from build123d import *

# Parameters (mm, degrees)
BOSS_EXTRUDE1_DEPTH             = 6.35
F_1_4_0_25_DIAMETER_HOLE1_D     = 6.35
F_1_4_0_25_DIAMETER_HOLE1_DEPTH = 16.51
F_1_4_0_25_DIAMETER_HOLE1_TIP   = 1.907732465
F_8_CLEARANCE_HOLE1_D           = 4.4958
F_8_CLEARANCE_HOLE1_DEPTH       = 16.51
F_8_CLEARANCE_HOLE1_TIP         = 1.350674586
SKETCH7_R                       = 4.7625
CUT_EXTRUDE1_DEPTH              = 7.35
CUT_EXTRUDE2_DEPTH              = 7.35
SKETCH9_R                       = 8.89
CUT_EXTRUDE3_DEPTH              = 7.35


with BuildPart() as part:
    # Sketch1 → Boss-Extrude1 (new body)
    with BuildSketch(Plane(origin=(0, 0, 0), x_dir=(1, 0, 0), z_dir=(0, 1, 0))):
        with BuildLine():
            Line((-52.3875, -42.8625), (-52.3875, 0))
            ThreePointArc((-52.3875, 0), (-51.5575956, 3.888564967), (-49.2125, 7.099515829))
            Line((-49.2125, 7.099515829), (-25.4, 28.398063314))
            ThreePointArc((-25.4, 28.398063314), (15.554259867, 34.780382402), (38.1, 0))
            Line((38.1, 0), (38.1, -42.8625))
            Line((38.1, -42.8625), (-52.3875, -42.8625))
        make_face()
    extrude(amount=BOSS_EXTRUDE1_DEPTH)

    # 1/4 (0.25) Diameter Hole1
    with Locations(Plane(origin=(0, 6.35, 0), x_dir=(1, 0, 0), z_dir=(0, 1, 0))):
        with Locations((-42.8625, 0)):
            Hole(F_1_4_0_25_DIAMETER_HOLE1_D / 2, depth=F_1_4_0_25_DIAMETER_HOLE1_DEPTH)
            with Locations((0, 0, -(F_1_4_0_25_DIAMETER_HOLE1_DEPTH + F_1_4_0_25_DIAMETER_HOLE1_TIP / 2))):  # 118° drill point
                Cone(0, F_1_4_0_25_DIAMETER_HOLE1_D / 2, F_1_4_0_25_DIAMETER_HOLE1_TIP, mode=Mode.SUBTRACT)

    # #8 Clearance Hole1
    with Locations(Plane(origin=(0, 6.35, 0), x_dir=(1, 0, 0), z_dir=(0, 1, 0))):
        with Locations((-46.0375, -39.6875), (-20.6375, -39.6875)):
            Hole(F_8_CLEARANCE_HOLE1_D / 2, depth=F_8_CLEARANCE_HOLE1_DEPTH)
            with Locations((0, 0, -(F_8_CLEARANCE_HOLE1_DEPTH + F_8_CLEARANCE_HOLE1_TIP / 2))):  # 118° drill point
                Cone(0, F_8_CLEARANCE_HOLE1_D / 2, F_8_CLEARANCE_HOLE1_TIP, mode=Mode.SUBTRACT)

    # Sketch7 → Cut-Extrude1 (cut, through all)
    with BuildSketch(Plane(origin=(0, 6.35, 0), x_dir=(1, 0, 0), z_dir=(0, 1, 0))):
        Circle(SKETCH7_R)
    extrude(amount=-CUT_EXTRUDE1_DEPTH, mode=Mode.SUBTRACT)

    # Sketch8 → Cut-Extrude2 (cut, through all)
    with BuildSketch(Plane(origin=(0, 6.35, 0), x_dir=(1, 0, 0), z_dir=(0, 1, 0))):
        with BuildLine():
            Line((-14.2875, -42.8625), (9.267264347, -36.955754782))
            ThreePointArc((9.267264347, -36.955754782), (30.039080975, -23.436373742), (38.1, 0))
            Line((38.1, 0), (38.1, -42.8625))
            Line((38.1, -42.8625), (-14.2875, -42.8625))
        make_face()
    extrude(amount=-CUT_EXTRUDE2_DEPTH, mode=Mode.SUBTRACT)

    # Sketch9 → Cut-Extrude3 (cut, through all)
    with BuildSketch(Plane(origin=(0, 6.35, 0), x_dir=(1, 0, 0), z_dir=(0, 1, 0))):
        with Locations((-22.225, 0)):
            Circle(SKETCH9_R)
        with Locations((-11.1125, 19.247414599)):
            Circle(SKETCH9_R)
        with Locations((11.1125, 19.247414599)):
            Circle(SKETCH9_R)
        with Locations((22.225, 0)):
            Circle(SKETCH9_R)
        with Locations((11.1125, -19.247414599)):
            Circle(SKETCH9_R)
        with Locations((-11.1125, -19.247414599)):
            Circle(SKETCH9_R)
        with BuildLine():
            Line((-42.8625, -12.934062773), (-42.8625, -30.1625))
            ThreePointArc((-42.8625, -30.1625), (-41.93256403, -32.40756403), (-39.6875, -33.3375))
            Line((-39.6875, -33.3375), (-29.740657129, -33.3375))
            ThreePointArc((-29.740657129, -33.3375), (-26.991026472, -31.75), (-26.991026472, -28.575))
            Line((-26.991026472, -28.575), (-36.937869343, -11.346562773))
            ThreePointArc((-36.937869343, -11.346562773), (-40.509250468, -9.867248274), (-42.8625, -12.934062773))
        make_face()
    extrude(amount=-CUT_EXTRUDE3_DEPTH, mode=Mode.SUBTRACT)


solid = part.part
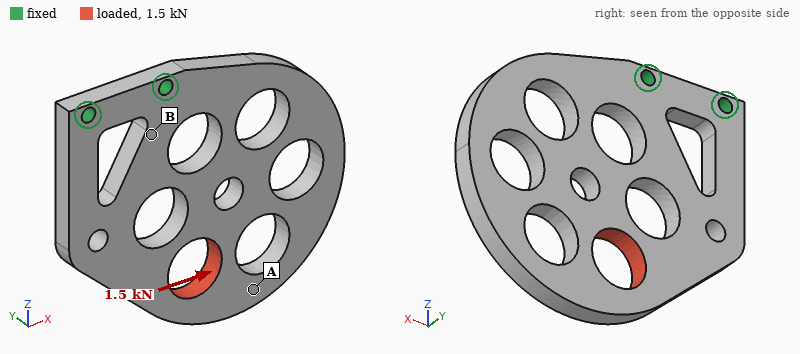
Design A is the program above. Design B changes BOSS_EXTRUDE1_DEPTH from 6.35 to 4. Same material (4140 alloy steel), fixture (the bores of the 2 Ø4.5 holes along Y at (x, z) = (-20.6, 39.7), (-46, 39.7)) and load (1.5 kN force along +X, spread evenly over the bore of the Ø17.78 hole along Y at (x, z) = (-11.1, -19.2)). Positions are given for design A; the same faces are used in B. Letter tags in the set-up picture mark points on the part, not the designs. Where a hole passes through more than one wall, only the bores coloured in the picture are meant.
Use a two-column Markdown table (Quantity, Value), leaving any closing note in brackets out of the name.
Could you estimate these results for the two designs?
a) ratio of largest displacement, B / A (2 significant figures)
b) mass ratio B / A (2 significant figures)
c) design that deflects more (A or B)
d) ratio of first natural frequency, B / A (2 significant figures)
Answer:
| Quantity | Value |
|---|---|
| ratio of largest displacement, B / A | 1.6 |
| mass ratio B / A | 0.63 |
| design that deflects more | B |
| ratio of first natural frequency, B / A | 0.66 |
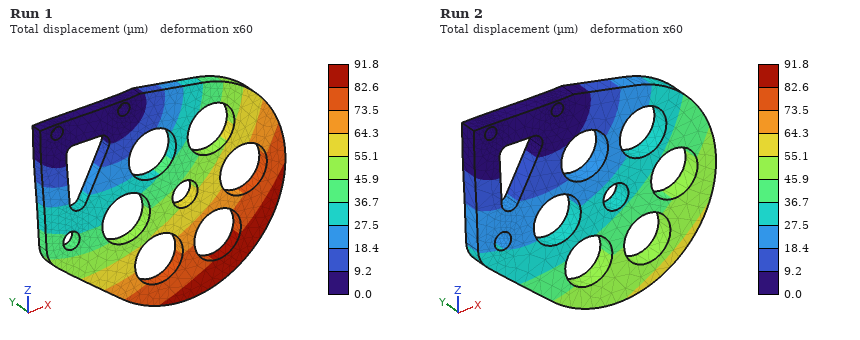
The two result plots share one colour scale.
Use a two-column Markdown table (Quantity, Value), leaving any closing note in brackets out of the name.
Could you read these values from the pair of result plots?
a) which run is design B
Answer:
| Quantity | Value |
|---|---|
| which run is design B | Run 1 |
